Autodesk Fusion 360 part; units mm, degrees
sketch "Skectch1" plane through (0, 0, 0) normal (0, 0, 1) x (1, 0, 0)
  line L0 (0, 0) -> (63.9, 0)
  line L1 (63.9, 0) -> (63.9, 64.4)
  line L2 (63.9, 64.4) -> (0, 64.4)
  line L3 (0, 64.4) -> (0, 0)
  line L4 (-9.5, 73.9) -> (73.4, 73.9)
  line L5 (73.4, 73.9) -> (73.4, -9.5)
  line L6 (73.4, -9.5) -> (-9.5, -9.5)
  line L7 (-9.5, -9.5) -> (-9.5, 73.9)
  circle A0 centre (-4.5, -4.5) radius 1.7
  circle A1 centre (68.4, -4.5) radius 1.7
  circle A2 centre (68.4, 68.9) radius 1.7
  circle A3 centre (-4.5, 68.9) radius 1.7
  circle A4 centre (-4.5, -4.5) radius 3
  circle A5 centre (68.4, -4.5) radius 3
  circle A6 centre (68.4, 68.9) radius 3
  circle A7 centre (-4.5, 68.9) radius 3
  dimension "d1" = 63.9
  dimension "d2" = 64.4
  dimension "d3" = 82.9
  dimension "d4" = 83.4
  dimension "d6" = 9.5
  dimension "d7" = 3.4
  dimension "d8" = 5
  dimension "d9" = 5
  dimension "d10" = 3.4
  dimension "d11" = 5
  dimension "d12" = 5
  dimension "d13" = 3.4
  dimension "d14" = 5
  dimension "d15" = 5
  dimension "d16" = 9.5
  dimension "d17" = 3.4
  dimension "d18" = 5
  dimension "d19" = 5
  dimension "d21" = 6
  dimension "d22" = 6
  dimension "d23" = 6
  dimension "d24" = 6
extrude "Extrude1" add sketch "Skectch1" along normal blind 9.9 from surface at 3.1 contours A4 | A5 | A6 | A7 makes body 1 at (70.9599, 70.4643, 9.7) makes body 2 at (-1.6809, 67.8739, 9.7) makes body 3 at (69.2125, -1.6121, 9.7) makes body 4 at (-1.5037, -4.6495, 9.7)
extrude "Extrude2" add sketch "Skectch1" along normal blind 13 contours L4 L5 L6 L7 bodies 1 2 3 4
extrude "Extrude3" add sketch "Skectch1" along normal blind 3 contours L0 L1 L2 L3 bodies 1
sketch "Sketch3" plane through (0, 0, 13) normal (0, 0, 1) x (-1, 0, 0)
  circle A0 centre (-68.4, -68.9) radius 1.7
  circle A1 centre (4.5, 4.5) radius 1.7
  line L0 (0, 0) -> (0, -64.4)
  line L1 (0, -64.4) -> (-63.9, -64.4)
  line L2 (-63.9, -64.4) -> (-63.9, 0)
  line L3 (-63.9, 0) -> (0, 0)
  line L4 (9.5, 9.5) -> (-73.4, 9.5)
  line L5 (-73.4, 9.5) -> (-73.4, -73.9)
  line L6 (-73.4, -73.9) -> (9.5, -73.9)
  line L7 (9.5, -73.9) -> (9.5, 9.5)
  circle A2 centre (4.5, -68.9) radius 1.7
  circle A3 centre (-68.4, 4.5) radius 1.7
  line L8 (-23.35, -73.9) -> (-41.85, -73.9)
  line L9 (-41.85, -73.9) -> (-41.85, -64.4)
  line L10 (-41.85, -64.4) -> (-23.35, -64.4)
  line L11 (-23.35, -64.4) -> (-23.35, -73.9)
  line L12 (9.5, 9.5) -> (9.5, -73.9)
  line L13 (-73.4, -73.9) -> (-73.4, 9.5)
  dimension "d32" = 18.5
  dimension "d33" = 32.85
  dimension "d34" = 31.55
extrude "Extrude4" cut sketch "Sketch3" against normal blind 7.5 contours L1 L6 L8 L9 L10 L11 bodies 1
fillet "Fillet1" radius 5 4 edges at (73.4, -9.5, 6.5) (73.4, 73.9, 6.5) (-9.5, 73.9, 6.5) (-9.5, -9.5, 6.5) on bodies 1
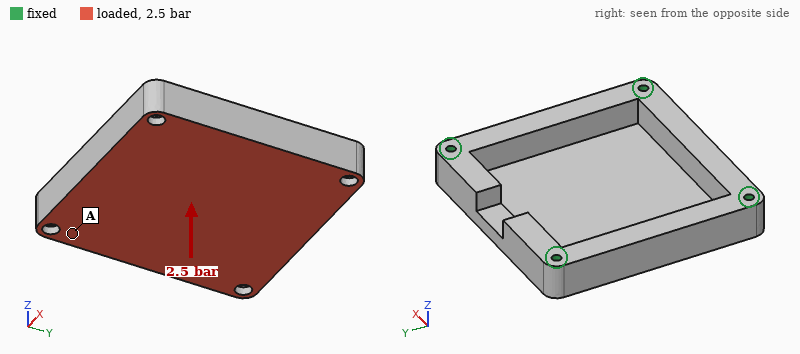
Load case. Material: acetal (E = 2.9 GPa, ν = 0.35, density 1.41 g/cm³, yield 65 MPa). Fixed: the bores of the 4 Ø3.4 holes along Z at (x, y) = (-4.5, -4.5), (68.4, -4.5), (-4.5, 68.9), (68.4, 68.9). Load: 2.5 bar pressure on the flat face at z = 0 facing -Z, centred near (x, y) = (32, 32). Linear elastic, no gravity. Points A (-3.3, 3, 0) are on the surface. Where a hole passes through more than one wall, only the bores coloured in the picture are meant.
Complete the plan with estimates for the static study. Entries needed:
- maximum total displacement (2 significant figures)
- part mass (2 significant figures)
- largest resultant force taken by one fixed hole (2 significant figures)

1.3 mm
65 g
650 N
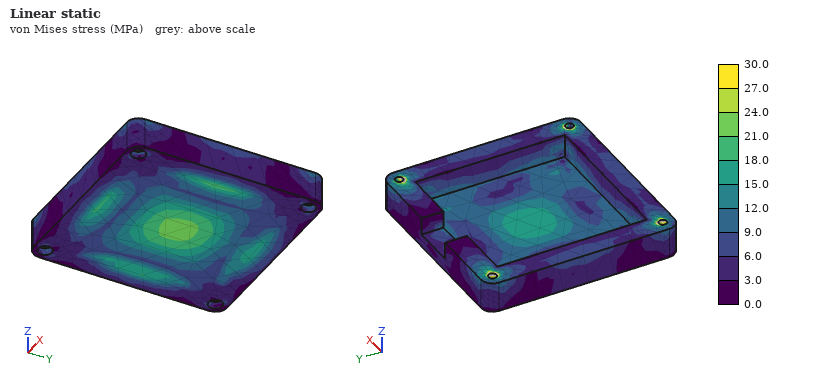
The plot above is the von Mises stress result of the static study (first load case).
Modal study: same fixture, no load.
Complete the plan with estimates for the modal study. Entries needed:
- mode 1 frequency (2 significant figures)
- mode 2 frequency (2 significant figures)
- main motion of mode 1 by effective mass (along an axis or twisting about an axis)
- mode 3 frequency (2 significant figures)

1400 Hz
2300 Hz
along Z
2300 Hz
